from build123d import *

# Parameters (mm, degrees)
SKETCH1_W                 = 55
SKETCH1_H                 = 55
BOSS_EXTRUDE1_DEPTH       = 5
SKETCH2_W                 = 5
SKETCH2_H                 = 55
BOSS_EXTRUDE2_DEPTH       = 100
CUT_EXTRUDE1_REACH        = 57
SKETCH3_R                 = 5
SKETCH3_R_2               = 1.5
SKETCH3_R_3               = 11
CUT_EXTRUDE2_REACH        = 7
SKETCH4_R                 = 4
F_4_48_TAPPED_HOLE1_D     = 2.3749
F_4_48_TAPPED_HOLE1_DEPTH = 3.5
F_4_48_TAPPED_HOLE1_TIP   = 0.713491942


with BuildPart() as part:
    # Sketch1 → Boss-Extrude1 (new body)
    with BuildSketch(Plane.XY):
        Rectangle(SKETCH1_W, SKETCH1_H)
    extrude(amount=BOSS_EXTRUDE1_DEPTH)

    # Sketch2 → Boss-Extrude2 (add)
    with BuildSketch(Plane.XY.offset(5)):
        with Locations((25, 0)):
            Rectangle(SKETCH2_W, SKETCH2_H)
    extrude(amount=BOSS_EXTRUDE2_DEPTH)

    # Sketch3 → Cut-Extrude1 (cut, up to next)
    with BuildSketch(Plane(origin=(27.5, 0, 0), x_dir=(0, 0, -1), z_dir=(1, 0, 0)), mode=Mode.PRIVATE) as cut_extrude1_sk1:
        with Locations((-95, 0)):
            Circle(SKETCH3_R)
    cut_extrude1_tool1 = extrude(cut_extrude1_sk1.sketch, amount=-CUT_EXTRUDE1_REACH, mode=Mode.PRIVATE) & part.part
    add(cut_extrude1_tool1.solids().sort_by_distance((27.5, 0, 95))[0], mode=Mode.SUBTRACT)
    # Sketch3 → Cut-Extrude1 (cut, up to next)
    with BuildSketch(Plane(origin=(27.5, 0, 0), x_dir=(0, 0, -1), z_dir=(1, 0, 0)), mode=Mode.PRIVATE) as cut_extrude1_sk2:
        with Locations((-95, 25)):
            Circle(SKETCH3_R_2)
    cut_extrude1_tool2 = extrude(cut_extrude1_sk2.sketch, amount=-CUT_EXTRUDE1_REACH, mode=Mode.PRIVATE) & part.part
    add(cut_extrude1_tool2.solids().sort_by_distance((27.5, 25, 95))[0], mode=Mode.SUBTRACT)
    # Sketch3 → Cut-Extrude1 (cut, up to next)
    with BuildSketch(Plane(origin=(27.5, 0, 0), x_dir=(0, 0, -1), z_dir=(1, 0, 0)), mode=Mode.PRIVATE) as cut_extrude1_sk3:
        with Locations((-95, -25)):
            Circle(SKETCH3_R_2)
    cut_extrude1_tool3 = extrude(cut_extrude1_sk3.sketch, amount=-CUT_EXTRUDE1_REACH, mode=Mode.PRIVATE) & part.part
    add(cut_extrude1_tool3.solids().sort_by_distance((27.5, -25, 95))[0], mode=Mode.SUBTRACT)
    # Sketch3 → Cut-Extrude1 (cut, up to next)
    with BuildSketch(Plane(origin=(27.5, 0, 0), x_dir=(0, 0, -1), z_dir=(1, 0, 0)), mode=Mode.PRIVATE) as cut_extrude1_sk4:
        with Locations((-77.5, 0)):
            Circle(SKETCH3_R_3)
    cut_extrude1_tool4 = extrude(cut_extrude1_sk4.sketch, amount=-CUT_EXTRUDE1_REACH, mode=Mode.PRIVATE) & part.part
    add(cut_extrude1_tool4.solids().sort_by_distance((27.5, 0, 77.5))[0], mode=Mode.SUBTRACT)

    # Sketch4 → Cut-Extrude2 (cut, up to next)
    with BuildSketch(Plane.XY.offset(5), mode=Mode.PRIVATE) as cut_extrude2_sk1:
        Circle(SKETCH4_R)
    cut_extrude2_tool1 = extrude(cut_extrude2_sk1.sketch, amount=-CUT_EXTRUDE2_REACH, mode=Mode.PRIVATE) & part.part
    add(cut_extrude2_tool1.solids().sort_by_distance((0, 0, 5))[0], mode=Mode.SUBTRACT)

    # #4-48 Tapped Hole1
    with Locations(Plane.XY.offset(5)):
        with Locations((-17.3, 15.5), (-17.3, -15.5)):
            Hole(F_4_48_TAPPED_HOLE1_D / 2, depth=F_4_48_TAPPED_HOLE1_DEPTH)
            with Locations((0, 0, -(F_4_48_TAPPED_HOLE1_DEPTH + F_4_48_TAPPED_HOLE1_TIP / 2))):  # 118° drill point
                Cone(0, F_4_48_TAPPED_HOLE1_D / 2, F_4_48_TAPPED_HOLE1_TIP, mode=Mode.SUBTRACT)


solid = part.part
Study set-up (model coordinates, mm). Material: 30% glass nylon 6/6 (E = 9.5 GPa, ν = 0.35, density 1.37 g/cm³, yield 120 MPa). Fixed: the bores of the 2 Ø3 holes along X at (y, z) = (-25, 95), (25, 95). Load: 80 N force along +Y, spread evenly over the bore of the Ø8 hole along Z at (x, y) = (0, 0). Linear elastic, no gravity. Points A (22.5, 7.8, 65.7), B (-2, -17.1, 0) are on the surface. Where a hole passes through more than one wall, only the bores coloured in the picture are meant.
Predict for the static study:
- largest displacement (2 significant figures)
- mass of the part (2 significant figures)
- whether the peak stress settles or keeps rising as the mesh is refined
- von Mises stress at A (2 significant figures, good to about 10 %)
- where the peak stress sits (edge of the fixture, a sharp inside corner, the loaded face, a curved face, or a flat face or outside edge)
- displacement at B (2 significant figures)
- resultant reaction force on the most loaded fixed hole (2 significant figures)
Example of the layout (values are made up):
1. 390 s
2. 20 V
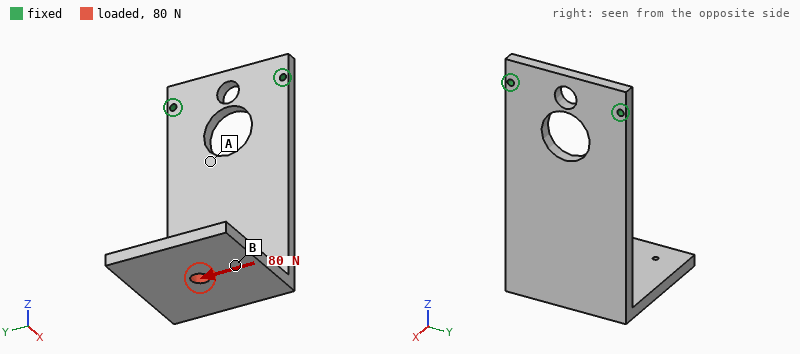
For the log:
1. 1.3 mm
2. 55 g
3. keeps rising
4. 8.2 MPa
5. edge of the fixture
6. 0.69 mm
7. 160 N
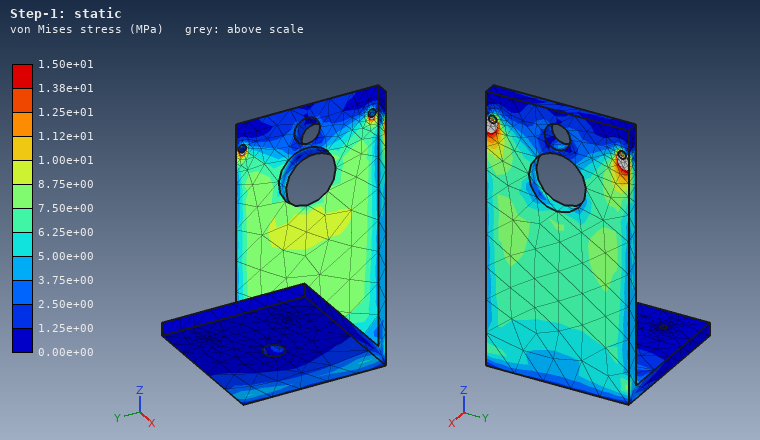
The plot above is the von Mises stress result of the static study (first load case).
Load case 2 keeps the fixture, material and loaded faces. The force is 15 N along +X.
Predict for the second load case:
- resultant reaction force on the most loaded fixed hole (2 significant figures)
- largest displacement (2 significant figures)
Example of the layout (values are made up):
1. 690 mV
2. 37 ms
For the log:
1. 7.5 N
2. 1.4 mm
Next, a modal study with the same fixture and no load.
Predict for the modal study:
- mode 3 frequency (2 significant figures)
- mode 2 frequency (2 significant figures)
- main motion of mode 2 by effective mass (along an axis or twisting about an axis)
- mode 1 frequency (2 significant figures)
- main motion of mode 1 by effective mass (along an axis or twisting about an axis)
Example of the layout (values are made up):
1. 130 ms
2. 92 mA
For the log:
1. 460 Hz
2. 310 Hz
3. along Y
4. 100 Hz
5. along X
